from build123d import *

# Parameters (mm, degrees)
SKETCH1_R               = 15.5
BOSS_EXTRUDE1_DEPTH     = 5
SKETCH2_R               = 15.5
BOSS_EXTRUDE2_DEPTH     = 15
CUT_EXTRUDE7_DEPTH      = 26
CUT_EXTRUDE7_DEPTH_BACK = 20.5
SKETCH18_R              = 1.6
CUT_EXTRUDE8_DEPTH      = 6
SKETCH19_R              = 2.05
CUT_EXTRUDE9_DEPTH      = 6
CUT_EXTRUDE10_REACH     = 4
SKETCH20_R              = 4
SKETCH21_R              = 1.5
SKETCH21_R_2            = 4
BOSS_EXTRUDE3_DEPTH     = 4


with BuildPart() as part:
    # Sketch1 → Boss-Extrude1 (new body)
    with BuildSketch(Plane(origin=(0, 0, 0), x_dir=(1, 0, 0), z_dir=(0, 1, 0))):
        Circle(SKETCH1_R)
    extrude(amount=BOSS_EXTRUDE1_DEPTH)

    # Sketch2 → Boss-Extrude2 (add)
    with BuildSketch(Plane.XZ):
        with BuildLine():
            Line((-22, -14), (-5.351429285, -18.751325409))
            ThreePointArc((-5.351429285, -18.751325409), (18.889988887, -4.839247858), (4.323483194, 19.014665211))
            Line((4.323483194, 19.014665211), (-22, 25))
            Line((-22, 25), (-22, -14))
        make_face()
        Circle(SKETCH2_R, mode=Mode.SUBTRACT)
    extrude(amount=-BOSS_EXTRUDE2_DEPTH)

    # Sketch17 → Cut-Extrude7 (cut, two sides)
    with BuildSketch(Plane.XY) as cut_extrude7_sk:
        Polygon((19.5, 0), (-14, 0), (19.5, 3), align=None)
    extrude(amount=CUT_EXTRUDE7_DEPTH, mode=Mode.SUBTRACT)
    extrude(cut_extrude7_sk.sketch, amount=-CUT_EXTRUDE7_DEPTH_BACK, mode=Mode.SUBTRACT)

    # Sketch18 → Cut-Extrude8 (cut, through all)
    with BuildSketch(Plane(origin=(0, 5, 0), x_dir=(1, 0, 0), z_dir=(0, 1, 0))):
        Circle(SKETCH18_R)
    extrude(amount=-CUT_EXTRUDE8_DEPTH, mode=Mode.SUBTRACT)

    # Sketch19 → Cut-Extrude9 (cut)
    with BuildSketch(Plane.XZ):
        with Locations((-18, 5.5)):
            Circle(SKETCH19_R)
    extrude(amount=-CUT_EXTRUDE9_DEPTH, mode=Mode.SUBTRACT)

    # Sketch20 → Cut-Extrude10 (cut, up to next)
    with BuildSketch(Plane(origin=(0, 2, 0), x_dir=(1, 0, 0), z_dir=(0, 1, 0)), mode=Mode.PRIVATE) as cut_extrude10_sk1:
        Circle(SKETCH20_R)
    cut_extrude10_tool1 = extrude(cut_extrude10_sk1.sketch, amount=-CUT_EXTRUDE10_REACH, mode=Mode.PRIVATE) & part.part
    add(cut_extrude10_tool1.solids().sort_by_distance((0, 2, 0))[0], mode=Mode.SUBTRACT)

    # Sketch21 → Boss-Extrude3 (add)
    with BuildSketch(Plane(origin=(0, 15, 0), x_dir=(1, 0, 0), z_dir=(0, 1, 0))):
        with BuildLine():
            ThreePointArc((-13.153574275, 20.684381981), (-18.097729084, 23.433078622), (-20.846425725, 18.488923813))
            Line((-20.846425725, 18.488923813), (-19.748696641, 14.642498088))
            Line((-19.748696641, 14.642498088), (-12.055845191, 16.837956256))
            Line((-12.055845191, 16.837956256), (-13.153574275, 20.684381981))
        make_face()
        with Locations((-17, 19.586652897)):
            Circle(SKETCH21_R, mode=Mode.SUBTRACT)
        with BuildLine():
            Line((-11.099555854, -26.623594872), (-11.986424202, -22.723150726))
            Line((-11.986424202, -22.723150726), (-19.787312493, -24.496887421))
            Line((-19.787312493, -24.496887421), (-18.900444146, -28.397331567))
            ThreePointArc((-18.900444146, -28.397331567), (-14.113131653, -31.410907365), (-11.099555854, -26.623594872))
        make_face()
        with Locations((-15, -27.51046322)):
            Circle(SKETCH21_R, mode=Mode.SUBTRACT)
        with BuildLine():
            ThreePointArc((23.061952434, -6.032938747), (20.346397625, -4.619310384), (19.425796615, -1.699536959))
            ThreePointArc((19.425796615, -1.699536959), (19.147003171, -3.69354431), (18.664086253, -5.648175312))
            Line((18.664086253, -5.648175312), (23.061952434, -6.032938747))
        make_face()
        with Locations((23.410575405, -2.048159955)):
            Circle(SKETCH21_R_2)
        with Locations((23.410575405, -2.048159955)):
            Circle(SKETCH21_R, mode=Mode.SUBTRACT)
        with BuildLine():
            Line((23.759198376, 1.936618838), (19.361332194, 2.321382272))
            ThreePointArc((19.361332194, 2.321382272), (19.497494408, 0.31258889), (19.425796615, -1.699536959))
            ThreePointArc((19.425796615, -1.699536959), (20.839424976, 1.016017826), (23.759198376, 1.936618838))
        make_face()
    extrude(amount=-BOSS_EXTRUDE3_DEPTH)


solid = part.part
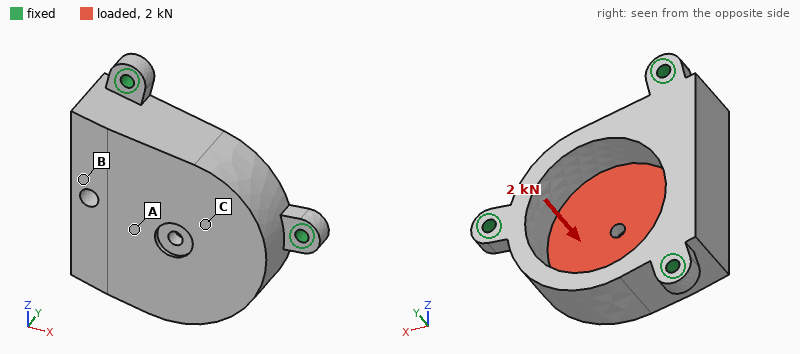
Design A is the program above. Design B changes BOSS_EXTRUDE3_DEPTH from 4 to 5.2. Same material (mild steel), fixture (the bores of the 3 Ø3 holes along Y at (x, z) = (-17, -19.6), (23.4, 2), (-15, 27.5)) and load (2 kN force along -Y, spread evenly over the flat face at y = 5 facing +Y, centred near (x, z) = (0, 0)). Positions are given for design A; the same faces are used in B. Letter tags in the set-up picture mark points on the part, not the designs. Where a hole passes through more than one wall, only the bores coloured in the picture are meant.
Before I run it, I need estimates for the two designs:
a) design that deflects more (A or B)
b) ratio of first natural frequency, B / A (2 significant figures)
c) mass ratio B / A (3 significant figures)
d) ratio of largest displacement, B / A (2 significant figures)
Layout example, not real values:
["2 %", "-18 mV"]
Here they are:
["A", "1.1", "1.01", "0.92"]
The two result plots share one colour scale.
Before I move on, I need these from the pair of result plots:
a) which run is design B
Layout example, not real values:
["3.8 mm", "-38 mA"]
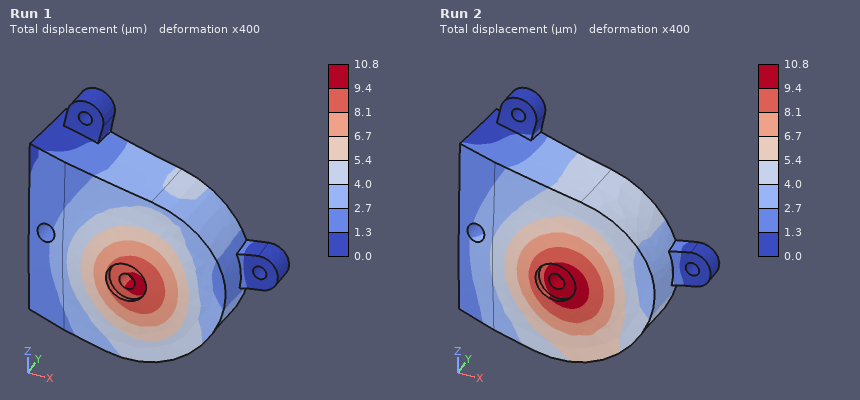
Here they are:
["Run 1"]
